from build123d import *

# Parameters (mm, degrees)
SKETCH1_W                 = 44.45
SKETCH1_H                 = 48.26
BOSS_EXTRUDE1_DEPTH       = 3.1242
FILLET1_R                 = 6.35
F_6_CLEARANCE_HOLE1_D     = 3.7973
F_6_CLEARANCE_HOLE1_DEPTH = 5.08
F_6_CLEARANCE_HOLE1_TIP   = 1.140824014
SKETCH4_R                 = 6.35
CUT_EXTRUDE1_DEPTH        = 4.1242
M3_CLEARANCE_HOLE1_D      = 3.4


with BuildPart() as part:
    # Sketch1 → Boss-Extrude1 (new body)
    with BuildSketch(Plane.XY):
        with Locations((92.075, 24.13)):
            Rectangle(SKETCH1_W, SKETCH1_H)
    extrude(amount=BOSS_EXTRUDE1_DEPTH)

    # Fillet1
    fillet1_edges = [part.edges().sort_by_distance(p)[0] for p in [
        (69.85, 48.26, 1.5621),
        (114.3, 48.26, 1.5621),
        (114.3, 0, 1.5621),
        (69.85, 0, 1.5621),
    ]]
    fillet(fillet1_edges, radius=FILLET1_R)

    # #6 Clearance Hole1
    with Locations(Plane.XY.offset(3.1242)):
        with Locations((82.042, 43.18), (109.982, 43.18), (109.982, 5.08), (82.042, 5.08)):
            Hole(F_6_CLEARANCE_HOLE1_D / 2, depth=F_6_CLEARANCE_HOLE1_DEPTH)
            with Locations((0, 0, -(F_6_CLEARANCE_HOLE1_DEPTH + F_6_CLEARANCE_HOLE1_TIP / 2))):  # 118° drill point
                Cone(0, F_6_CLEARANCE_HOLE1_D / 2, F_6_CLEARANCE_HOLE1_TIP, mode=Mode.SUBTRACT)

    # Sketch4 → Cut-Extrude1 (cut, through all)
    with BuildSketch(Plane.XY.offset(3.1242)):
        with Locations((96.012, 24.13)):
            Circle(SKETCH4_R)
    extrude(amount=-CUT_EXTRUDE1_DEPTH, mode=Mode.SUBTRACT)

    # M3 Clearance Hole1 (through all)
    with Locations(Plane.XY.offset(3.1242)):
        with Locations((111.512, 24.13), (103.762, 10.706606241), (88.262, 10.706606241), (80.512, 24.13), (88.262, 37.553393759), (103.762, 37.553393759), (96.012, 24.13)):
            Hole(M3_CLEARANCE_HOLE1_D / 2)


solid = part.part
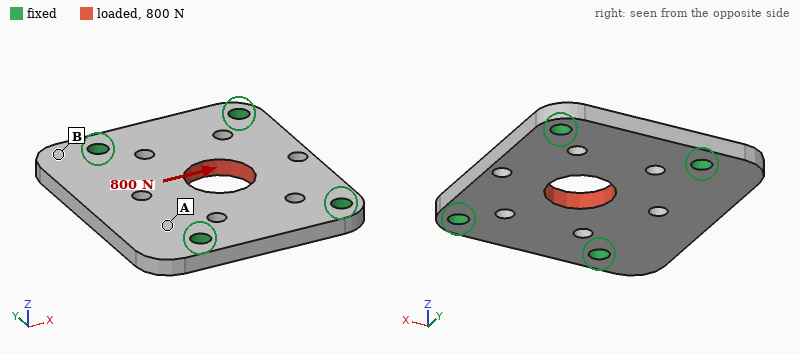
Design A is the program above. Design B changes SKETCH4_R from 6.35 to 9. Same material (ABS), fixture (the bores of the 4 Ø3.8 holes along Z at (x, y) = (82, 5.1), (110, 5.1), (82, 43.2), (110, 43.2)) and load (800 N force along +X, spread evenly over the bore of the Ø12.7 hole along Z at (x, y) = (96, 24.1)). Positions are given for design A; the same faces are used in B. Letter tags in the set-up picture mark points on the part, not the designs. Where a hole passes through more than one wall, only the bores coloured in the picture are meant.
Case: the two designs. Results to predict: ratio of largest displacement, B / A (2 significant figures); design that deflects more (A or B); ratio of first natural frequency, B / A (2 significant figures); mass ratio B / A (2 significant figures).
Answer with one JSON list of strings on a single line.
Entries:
["1.1", "B", "1.0", "0.93"]
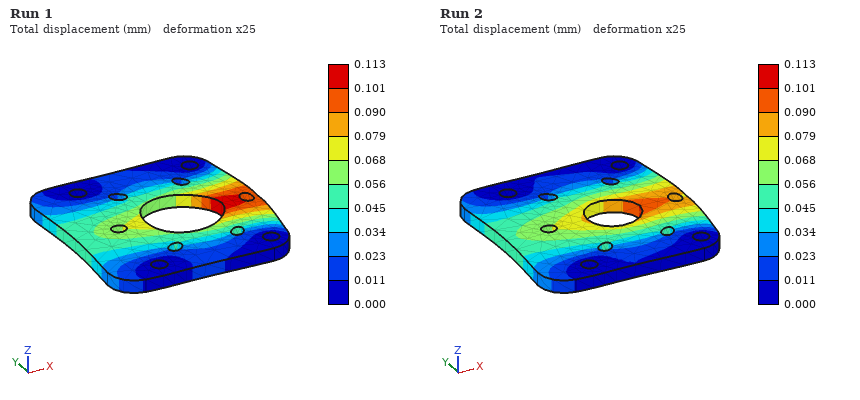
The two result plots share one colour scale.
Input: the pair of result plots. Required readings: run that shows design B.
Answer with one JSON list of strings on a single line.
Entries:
["Run 1"]
